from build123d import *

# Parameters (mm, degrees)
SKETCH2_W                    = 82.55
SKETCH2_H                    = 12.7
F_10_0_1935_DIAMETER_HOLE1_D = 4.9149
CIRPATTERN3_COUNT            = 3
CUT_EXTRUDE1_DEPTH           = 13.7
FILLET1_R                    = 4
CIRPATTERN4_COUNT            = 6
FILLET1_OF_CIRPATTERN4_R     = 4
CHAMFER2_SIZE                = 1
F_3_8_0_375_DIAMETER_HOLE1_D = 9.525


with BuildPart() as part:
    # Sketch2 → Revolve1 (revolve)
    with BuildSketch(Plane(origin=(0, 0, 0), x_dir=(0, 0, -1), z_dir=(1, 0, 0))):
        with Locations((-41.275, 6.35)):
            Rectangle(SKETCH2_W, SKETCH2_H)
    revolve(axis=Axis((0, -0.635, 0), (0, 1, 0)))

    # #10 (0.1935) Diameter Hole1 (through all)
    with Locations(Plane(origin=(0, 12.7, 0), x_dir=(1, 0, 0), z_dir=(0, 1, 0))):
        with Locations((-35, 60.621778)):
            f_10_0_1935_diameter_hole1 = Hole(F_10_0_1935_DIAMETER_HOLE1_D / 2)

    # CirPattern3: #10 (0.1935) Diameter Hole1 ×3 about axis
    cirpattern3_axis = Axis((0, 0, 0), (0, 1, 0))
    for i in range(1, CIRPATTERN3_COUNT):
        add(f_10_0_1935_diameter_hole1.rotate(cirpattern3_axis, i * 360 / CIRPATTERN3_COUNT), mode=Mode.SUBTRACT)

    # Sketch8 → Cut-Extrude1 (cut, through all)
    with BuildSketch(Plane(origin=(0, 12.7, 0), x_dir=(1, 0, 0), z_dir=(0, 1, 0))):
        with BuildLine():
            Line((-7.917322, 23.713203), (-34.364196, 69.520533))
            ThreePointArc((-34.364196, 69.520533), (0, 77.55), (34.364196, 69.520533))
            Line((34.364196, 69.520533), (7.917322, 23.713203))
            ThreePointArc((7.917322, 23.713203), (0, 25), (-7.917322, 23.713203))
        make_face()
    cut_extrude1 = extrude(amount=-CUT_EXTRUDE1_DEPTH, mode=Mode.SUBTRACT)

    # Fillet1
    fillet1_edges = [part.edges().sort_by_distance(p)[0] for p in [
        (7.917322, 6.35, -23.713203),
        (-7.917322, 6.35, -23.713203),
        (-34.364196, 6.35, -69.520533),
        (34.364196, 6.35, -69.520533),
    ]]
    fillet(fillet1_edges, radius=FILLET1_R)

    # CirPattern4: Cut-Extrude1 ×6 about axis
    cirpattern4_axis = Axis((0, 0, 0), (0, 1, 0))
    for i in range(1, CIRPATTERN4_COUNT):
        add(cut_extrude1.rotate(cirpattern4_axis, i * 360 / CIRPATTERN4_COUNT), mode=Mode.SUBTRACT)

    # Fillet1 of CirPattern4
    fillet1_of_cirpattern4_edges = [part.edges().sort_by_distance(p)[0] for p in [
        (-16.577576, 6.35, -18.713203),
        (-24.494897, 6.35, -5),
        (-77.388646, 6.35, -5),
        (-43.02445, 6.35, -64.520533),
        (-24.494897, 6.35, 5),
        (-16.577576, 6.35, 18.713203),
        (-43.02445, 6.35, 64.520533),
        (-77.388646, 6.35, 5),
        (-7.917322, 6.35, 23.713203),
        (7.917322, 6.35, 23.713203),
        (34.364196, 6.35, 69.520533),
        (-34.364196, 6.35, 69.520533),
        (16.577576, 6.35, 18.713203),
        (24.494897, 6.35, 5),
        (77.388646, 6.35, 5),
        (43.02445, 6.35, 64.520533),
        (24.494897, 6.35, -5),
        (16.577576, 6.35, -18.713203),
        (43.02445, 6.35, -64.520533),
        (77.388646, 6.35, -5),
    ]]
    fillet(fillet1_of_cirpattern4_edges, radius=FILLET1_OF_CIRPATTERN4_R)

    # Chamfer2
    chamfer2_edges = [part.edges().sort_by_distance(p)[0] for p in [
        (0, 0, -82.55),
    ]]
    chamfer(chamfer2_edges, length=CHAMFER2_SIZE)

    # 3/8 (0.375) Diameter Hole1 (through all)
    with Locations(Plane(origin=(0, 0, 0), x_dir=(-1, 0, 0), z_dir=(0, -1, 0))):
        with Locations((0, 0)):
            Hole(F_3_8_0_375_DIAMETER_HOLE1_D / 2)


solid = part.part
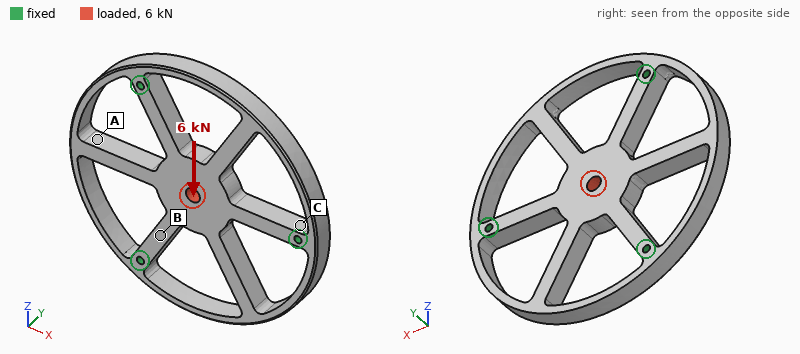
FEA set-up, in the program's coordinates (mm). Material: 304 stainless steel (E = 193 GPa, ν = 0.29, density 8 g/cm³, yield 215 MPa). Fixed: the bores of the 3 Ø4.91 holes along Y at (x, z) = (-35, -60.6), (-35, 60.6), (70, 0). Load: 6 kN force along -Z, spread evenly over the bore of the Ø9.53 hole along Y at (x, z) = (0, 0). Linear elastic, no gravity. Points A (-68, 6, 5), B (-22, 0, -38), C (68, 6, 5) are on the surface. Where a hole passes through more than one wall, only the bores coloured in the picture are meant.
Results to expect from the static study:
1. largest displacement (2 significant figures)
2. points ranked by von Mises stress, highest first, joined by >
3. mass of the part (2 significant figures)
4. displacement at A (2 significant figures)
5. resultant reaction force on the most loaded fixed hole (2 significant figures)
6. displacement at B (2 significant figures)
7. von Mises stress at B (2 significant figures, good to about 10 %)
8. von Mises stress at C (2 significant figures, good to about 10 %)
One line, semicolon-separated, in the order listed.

9.6 µm; B > C > A; 770 g; 3.9 µm; 3.2 kN; 4.0 µm; 25 MPa; 14 MPa
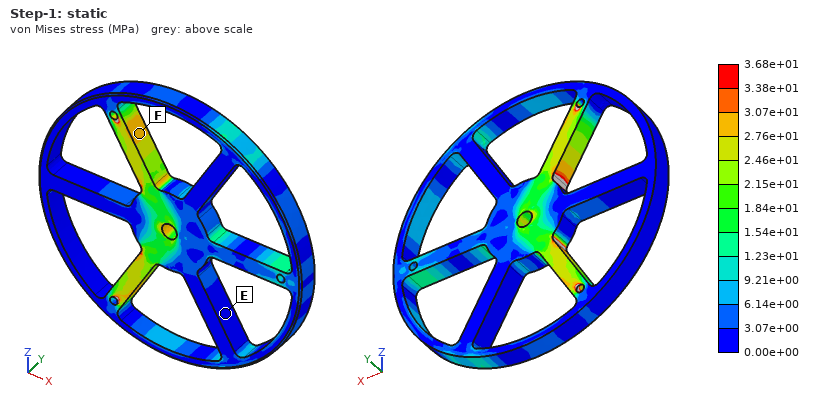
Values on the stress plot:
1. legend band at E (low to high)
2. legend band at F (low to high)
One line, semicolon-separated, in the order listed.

0.00e+00 to 3.07e+00 MPa; 2.76e+01 to 3.07e+01 MPa
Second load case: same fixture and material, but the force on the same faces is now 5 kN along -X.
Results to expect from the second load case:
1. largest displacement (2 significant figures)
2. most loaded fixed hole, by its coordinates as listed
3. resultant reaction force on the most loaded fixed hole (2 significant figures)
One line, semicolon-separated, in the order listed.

8.0 µm; (70, 0); 3.1 kN
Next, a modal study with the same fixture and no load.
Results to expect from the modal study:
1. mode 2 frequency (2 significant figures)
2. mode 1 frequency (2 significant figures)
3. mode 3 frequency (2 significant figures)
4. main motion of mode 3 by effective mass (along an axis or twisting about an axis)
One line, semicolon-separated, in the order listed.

1700 Hz; 1700 Hz; 1900 Hz; along Y
